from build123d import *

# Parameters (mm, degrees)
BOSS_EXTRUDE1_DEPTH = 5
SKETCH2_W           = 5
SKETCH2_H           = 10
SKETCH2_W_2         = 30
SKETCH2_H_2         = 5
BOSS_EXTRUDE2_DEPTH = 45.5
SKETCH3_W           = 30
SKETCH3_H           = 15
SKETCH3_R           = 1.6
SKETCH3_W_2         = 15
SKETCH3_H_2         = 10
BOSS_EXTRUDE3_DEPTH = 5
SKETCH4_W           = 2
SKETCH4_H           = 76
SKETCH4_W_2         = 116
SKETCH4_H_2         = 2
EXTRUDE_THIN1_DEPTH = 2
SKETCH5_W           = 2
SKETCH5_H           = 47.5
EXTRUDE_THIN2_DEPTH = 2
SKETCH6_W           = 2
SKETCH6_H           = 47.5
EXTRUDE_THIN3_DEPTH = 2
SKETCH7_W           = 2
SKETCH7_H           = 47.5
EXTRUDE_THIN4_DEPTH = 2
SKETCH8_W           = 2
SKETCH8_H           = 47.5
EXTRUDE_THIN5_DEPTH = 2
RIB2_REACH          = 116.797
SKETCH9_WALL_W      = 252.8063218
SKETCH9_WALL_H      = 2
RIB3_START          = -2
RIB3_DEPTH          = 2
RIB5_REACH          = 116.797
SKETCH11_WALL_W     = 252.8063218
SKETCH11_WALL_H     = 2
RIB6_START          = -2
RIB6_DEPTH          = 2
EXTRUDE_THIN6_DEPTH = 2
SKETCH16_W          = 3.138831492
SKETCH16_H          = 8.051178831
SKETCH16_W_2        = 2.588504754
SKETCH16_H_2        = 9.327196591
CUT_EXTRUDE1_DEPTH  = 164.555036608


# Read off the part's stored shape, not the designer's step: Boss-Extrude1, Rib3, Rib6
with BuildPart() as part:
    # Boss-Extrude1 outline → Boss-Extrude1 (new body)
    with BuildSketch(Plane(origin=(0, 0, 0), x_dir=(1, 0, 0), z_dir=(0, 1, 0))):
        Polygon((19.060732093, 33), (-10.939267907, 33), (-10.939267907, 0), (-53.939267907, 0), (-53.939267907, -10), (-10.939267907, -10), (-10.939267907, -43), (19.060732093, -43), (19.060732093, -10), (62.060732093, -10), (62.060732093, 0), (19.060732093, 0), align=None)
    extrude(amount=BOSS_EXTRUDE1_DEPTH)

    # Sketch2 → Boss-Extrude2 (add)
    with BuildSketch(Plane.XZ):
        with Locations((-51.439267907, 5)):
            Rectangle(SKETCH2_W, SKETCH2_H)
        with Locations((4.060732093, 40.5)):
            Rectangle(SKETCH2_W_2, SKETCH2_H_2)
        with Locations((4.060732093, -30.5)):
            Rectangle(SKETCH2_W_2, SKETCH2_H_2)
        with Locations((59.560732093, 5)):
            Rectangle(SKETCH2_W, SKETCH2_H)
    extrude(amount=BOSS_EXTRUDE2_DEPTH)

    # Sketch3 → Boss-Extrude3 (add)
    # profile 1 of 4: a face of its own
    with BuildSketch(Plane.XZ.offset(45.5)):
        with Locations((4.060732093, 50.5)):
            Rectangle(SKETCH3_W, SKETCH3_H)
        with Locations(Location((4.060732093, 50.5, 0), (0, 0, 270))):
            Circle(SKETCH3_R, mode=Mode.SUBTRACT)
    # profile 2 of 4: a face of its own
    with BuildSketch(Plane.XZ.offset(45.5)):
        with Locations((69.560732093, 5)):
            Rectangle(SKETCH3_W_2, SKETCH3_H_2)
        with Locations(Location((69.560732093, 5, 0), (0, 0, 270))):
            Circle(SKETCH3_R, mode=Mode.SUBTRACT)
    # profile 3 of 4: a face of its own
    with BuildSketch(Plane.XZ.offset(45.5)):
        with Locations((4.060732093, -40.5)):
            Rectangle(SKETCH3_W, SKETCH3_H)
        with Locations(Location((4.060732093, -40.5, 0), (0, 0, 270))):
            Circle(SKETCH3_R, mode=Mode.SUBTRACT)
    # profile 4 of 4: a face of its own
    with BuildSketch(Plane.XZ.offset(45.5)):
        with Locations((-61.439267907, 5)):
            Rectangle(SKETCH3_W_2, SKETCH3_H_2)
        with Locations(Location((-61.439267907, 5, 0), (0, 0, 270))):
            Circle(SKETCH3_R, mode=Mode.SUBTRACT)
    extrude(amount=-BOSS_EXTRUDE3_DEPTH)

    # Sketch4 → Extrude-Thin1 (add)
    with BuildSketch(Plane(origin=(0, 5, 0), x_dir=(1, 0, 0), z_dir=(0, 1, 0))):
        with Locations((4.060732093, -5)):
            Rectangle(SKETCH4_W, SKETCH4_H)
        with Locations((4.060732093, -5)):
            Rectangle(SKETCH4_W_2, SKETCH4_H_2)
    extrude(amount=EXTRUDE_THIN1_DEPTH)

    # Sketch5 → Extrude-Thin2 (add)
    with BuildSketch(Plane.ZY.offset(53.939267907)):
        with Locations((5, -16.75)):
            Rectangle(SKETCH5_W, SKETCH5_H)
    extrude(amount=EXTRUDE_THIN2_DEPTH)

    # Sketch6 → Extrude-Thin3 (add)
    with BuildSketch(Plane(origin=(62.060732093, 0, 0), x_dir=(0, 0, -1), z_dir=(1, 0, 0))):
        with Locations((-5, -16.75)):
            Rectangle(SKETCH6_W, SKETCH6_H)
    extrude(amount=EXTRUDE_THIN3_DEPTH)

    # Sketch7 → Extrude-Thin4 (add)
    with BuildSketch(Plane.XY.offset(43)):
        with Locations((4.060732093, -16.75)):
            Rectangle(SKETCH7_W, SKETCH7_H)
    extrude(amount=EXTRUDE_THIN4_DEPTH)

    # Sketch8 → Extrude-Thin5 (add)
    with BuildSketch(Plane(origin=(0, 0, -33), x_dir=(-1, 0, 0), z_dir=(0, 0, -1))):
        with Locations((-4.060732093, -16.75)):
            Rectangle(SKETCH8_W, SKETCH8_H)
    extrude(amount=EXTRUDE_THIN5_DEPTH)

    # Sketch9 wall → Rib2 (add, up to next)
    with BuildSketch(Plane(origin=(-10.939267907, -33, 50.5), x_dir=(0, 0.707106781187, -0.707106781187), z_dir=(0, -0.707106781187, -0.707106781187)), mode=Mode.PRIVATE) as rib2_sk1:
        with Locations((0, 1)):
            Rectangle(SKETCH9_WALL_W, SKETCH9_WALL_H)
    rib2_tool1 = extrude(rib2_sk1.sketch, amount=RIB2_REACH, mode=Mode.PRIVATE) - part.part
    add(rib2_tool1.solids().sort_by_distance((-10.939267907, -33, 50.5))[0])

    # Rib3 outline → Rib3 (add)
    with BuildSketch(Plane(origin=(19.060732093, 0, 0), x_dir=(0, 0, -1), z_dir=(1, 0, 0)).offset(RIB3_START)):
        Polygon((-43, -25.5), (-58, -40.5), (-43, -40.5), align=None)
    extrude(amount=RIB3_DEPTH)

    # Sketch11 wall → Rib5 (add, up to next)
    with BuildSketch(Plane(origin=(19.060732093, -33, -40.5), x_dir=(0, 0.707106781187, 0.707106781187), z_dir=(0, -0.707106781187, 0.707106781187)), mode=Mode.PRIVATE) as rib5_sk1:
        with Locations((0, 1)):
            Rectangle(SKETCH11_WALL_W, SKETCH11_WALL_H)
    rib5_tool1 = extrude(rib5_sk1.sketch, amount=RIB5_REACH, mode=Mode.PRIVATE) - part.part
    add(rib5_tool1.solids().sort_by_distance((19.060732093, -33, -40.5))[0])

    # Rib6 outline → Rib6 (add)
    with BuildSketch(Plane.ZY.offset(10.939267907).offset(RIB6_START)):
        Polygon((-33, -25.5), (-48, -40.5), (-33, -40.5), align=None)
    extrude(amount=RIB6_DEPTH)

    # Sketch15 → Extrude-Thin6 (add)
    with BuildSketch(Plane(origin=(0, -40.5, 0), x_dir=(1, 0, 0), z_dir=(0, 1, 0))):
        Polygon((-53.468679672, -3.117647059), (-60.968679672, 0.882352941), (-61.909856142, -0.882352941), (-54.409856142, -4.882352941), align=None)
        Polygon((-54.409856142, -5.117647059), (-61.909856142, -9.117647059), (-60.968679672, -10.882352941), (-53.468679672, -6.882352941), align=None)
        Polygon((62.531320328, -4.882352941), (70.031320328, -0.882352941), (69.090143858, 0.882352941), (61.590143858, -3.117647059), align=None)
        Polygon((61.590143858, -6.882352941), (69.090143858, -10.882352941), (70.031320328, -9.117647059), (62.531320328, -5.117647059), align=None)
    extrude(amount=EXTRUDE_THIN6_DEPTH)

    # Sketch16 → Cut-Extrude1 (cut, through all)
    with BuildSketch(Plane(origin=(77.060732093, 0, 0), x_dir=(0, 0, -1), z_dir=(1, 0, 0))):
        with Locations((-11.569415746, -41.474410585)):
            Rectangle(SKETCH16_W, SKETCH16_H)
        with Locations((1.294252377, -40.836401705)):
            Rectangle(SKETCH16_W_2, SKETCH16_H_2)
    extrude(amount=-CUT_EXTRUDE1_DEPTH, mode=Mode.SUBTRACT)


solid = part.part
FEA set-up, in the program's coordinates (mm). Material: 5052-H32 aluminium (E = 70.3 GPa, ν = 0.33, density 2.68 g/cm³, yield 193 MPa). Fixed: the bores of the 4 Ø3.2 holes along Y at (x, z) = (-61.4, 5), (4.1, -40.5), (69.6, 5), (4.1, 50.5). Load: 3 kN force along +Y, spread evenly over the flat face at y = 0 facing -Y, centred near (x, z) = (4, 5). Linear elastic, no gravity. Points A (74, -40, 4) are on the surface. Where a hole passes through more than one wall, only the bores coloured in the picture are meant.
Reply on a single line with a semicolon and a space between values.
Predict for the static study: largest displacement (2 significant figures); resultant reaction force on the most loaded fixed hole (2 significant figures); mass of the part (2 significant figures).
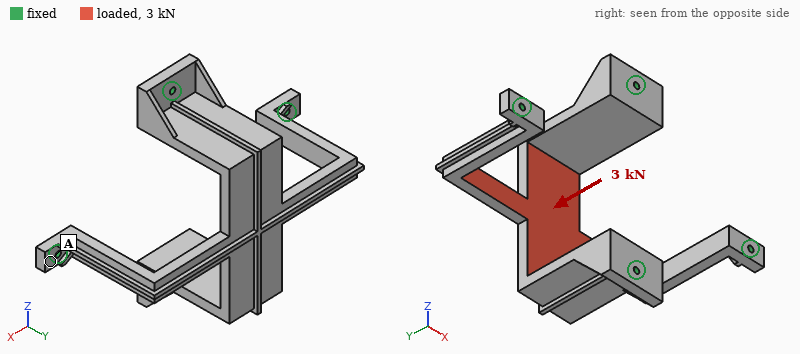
0.17 mm; 1.2 kN; 110 g
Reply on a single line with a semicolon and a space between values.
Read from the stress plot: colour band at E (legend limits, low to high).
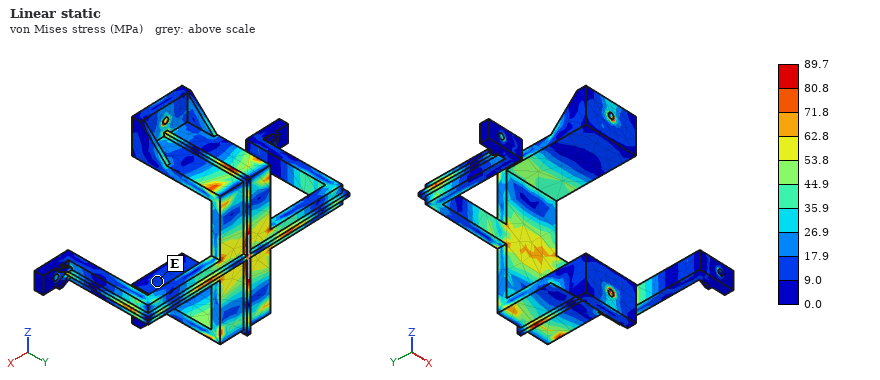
9.0 to 17.9 MPa
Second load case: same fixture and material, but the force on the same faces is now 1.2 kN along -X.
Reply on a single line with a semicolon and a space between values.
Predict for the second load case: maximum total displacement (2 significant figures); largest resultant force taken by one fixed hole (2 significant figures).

0.25 mm; 420 N
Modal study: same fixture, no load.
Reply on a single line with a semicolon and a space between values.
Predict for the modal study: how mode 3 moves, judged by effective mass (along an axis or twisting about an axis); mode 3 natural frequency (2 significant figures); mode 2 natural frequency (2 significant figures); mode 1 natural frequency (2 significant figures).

twisting about Y; 2000 Hz; 1500 Hz; 1400 Hz
